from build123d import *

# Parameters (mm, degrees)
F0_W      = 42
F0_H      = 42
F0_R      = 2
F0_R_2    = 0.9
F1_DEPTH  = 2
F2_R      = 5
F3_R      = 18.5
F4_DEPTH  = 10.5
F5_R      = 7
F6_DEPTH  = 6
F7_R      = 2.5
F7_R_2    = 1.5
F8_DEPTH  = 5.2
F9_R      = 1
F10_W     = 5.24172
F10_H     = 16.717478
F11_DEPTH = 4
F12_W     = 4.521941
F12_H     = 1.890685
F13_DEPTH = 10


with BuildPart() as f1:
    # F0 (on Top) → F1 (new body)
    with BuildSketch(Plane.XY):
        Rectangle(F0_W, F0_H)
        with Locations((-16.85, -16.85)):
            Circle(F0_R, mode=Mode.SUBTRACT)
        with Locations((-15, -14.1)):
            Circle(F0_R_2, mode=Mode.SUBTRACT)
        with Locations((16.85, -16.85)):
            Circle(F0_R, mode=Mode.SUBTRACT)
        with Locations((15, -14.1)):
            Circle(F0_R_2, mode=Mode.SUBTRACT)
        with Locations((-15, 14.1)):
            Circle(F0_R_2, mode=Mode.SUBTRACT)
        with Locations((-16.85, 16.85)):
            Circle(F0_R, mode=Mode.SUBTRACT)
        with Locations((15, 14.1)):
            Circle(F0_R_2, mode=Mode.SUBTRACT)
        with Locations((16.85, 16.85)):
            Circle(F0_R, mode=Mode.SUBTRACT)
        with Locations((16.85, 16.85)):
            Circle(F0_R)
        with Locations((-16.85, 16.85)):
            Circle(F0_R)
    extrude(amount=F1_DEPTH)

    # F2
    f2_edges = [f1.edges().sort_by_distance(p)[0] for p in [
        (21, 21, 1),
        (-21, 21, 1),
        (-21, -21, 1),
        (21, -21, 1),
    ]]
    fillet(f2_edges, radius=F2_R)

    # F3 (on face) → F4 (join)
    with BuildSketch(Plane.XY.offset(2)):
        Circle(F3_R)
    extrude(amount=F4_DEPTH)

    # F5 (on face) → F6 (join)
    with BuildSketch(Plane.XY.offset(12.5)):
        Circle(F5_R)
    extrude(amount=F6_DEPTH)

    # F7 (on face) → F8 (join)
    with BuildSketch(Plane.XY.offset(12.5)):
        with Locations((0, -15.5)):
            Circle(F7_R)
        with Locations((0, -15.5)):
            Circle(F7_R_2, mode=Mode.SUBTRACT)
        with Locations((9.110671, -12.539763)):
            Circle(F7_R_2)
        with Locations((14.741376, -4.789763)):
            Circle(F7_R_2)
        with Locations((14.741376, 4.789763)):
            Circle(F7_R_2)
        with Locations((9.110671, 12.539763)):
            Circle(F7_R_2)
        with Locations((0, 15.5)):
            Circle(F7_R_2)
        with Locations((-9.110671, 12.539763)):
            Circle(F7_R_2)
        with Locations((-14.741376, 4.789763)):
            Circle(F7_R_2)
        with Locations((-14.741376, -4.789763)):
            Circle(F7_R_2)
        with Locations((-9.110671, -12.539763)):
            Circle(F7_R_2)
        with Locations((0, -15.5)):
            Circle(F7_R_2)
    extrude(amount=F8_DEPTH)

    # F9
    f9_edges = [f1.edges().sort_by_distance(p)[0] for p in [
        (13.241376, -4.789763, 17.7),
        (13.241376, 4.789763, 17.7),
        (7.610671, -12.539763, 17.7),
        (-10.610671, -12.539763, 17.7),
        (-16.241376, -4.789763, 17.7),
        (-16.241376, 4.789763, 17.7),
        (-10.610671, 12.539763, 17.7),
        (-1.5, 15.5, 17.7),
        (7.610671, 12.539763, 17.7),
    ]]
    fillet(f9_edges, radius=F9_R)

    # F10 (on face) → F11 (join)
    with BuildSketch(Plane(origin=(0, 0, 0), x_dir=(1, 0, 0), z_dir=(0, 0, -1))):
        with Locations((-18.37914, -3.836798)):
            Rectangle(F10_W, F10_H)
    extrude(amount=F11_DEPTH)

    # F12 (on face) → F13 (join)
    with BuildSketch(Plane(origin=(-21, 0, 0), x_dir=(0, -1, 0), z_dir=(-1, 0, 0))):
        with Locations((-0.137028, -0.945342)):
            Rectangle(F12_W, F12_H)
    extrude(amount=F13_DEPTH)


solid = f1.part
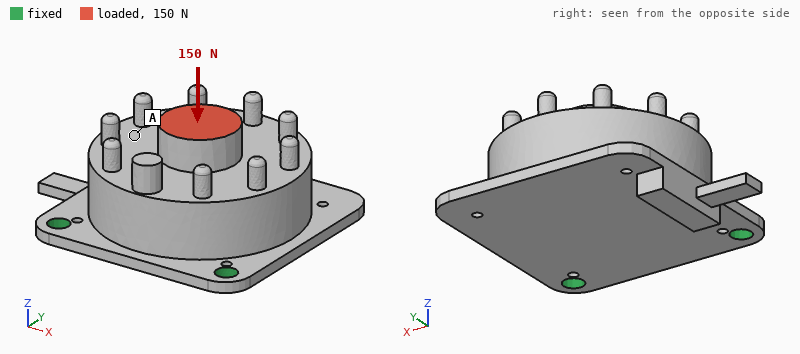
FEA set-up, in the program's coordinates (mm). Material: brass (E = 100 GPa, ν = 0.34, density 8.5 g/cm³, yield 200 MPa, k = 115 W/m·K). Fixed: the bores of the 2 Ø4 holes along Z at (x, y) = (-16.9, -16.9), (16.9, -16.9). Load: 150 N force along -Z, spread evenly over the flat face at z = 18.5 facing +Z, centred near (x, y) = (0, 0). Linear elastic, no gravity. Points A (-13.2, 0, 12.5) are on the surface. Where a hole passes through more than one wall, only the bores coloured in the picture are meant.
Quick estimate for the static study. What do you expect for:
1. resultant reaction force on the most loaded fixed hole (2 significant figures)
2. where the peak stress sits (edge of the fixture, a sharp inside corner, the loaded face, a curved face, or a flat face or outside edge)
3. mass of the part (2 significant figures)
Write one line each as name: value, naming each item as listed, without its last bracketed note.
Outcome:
resultant reaction force on the most loaded fixed hole: 75 N
where the peak stress sits: a curved face
mass of the part: 140 g
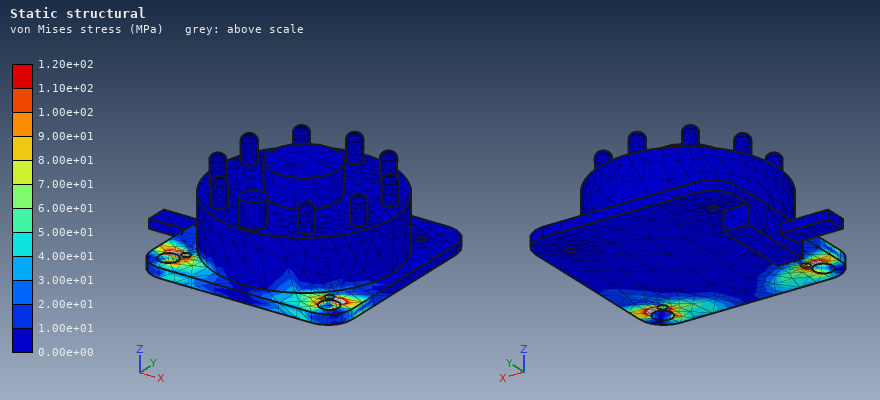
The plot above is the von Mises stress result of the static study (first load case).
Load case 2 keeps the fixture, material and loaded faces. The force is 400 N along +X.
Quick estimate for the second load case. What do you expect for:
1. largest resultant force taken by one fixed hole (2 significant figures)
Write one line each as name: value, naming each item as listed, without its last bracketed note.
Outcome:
largest resultant force taken by one fixed hole: 360 N
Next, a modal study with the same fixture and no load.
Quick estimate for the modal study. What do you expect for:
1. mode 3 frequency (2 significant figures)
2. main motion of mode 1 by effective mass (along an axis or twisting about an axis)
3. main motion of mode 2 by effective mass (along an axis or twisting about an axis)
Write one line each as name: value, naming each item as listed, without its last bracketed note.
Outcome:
mode 3 frequency: 5600 Hz
main motion of mode 1 by effective mass: along Z
main motion of mode 2 by effective mass: along X
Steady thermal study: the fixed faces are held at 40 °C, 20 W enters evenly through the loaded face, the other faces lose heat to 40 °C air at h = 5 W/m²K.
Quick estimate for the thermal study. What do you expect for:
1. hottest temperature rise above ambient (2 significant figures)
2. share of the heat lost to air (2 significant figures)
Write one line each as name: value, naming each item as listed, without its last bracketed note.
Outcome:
hottest temperature rise above ambient: 37 K
share of the heat lost to air: 3.6 %
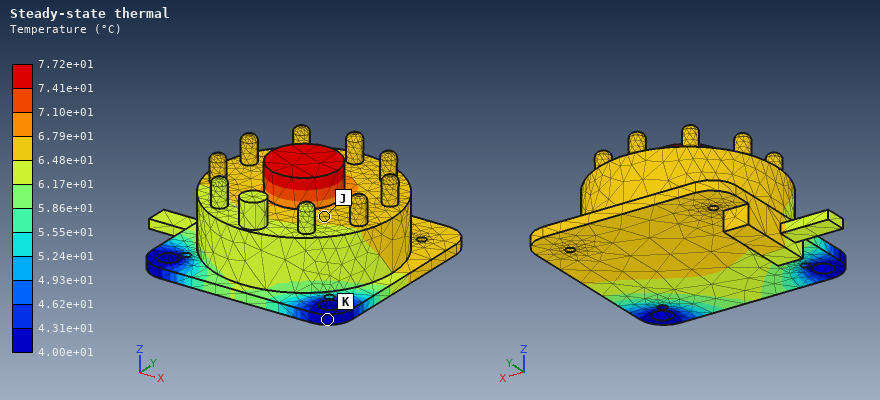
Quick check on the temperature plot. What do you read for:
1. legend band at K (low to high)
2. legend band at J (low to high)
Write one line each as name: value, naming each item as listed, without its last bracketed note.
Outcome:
legend band at K: 4.00e+01 to 4.31e+01 °C
legend band at J: 6.48e+01 to 6.79e+01 °C
